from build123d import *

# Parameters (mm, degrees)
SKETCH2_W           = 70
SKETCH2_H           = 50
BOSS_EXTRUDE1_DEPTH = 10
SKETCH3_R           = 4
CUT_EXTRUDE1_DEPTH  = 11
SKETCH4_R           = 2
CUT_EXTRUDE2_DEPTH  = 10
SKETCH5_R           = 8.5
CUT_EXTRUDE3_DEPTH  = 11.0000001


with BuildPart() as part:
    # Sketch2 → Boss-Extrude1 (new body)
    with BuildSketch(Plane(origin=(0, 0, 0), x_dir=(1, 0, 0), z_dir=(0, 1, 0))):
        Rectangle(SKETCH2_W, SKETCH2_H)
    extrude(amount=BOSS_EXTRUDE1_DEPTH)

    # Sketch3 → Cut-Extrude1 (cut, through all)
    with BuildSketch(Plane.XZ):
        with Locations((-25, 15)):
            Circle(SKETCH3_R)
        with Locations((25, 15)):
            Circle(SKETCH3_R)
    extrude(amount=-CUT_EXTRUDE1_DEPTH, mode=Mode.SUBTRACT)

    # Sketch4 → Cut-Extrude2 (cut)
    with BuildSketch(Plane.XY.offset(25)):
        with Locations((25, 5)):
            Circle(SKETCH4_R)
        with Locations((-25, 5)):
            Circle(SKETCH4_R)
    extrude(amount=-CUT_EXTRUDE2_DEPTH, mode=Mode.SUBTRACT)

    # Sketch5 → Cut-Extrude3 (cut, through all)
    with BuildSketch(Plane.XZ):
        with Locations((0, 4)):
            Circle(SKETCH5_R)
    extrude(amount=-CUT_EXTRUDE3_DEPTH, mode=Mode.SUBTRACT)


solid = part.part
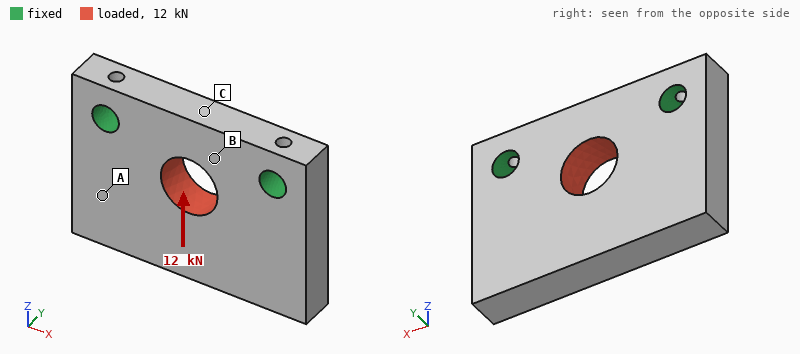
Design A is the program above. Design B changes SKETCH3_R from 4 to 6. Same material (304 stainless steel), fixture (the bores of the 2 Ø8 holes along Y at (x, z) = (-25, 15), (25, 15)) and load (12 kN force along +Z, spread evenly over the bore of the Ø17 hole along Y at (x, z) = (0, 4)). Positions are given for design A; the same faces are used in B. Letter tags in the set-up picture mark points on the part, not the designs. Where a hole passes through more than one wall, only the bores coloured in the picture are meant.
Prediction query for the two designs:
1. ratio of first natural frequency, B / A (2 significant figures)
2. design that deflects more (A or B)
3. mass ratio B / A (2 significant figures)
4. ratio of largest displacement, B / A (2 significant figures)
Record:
1.1
A
0.96
0.83
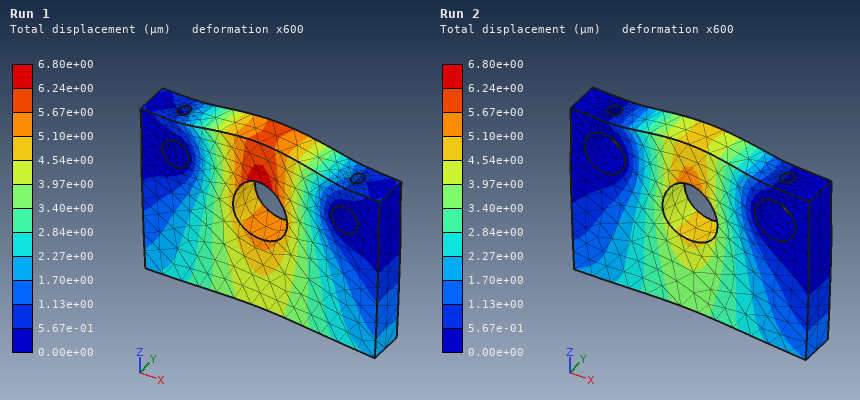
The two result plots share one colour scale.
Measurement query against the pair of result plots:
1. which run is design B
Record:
Run 2
